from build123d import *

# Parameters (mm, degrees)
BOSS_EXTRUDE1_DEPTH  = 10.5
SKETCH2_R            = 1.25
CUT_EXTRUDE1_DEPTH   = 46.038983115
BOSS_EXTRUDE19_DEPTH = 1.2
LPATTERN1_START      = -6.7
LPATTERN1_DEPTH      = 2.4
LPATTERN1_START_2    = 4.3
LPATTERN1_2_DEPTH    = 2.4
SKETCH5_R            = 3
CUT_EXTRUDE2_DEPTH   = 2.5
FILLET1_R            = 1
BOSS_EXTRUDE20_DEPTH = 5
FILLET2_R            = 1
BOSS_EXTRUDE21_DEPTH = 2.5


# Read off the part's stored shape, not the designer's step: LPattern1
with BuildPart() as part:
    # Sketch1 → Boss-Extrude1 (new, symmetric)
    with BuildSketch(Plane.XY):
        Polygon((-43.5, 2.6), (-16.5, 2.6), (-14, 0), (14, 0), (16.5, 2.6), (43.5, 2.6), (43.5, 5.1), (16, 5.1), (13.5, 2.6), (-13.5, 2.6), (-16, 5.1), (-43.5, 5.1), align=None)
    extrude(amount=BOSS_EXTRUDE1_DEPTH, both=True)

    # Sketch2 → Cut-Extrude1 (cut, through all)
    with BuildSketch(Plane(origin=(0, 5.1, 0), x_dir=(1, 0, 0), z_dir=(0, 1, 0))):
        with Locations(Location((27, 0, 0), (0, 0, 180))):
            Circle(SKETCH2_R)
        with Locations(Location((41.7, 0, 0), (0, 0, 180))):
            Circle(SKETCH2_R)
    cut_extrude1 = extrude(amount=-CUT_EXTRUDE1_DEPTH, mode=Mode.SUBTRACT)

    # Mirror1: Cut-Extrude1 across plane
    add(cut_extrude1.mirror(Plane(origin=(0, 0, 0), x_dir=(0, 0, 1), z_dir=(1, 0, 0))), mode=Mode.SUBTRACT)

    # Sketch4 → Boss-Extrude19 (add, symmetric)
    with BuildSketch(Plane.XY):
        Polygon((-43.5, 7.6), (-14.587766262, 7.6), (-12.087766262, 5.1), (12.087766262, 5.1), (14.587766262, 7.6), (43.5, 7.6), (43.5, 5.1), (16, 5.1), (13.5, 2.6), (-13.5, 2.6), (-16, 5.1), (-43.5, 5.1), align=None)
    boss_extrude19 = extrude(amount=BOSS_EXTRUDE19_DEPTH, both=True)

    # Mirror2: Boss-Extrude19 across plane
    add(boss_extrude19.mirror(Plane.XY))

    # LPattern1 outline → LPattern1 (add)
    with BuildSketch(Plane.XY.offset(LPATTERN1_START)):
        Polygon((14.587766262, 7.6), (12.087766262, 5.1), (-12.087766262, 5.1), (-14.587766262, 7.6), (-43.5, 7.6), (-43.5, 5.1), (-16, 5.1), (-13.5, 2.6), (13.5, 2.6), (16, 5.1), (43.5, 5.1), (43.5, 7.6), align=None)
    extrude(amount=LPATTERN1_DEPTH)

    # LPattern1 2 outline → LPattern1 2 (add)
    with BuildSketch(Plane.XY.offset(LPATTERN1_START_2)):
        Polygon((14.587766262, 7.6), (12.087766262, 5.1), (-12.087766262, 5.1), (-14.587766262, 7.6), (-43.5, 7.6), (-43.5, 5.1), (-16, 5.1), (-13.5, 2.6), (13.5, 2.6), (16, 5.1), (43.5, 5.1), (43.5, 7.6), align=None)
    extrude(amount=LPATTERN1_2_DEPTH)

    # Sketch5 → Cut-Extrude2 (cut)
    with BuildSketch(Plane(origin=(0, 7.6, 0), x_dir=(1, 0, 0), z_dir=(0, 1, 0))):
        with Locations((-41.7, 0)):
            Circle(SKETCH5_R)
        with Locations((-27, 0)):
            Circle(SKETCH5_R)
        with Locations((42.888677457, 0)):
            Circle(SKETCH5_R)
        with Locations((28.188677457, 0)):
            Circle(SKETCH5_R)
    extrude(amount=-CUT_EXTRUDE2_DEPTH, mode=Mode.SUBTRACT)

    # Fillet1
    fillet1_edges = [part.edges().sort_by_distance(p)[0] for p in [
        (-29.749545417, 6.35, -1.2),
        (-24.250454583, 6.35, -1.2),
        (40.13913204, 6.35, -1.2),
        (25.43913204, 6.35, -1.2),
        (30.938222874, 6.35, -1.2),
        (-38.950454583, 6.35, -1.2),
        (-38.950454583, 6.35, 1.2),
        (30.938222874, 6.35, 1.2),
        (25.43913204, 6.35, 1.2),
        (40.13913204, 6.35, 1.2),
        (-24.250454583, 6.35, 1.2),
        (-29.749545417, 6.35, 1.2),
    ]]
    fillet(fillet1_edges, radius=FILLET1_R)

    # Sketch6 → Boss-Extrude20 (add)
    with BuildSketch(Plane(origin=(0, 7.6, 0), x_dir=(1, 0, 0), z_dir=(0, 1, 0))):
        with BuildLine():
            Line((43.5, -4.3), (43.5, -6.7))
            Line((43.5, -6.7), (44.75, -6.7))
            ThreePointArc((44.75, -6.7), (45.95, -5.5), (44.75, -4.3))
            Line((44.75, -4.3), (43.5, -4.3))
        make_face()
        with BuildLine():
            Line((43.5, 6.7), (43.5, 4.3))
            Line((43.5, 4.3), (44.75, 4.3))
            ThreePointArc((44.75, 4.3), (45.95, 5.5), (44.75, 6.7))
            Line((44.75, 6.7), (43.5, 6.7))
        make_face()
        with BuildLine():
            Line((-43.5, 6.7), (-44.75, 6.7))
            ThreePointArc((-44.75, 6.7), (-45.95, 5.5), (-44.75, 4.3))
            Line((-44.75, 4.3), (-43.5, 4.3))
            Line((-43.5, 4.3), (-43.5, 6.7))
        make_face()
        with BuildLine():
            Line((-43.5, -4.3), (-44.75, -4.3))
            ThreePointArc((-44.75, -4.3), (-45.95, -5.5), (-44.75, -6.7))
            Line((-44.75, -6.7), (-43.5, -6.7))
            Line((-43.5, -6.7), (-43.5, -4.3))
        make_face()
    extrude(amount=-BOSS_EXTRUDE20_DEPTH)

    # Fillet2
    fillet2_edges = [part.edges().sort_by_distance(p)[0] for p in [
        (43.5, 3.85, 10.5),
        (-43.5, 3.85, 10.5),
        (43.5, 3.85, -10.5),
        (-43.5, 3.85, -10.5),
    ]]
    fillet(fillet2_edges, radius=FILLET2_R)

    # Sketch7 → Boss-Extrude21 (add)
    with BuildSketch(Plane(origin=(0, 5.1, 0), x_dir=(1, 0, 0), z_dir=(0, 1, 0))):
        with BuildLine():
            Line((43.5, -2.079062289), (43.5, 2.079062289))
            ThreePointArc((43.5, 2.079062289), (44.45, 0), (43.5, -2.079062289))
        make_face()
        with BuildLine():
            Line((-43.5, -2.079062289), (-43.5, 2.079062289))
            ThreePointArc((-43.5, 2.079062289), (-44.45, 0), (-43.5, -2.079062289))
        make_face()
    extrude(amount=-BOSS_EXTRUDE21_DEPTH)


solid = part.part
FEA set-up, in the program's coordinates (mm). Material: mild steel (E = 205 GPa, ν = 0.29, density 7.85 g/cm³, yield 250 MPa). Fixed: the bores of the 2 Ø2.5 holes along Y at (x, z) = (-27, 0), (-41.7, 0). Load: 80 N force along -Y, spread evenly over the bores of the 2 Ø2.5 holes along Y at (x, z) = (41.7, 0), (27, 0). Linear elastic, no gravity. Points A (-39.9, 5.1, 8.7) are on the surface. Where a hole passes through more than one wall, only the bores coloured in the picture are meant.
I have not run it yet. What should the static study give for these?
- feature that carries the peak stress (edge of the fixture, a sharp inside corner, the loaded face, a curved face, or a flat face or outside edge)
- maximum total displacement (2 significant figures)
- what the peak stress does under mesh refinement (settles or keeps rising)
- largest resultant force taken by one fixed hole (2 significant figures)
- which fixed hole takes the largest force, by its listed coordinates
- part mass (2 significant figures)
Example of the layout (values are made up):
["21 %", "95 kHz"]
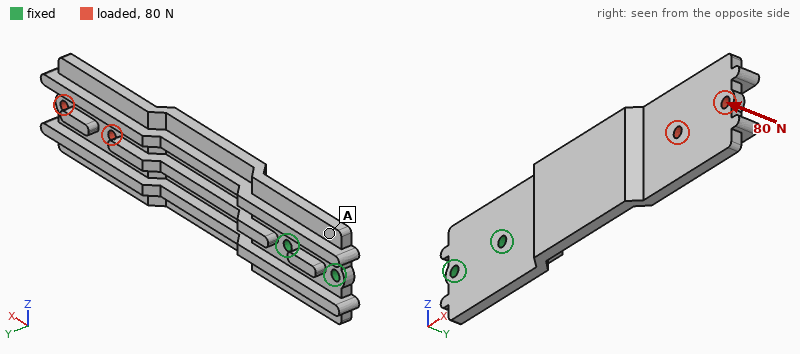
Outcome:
["edge of the fixture", "0.41 mm", "keeps rising", "350 N", "(-27, 0)", "49 g"]
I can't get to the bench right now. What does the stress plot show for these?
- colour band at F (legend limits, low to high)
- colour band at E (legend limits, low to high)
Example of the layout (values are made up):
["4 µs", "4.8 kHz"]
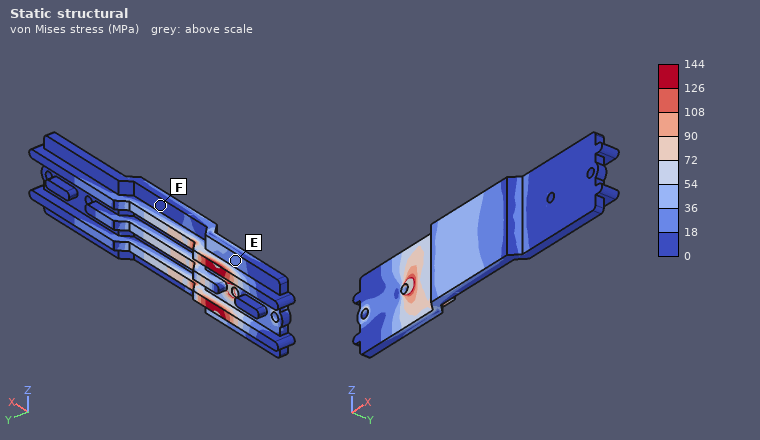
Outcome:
["0 to 18 MPa", "18 to 36 MPa"]
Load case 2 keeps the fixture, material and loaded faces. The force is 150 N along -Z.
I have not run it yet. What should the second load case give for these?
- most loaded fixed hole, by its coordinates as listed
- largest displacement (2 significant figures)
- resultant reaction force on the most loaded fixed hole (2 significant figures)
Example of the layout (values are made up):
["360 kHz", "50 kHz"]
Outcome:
["(-27, 0)", "81 µm", "690 N"]
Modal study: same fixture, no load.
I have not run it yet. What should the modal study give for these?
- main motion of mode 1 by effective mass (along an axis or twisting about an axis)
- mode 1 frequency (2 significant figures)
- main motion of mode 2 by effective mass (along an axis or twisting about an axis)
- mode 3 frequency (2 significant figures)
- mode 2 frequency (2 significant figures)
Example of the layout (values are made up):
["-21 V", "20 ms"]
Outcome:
["along Y", "640 Hz", "along Z", "3100 Hz", "1900 Hz"]
